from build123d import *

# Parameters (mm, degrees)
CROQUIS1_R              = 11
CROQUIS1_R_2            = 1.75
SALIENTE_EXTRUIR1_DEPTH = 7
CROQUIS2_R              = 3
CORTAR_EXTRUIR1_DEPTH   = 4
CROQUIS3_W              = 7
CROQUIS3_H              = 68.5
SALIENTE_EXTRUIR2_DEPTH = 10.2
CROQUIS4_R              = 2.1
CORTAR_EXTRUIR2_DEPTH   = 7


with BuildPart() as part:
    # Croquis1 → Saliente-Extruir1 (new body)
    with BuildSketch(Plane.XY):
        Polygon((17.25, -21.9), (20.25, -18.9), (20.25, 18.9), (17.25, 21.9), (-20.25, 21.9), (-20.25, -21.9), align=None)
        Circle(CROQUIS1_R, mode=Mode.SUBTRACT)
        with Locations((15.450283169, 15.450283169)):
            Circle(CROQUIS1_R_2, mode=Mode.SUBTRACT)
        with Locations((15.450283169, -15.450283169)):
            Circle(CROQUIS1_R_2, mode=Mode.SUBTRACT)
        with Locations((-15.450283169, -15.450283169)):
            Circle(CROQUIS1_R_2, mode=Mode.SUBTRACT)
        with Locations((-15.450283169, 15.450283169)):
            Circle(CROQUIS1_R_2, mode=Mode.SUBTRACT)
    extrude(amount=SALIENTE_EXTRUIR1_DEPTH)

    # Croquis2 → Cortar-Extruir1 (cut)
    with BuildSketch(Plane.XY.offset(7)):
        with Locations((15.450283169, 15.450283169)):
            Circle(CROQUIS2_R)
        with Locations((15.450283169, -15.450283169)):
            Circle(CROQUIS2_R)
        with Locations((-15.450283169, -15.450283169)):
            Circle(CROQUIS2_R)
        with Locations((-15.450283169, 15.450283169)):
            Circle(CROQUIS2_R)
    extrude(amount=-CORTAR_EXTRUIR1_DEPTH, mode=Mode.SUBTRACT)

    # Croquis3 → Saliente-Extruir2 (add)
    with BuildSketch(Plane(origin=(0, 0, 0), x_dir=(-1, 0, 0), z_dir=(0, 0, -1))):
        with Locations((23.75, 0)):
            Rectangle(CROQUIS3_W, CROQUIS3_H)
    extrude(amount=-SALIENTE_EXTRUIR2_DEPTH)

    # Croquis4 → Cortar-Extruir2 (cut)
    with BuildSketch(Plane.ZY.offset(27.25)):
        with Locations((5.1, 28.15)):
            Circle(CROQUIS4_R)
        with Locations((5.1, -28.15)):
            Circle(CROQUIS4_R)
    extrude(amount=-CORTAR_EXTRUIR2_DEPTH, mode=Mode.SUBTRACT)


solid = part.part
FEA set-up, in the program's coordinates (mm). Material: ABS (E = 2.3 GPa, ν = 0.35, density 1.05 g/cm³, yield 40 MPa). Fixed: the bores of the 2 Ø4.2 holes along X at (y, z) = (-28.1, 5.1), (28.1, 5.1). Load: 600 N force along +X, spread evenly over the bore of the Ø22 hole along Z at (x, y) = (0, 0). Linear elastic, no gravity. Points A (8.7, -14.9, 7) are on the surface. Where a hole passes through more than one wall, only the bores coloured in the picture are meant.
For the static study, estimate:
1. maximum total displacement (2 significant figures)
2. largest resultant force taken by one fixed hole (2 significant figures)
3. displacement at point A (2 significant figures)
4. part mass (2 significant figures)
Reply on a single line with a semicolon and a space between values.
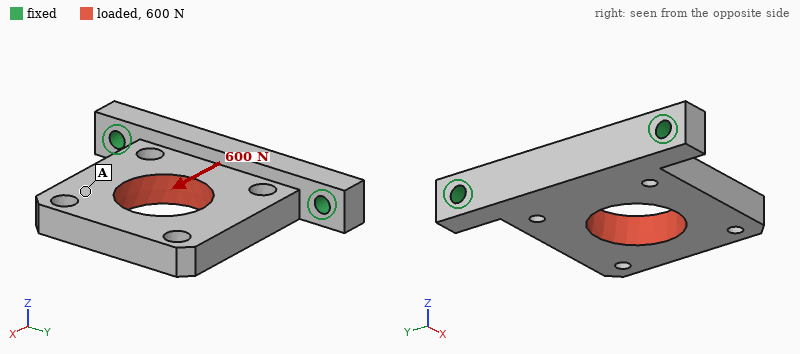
0.27 mm; 330 N; 0.20 mm; 15 g
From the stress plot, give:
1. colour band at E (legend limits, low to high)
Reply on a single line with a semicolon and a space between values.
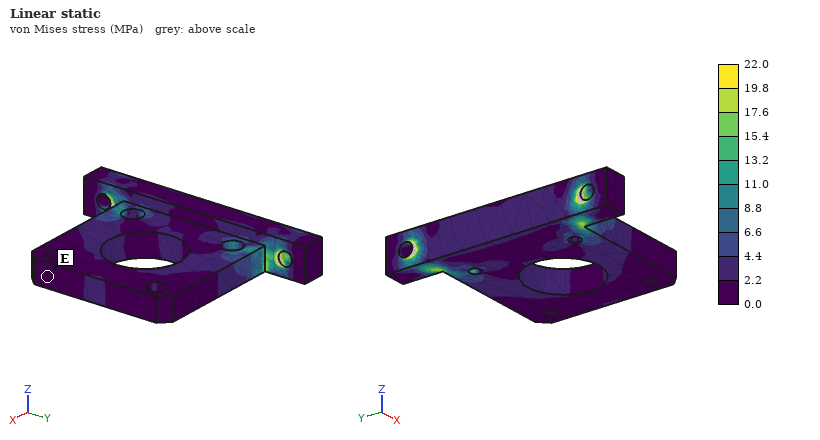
0.0 to 2.2 MPa
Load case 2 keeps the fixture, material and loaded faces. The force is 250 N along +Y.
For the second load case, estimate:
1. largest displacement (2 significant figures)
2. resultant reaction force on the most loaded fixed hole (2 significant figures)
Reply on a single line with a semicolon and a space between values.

0.17 mm; 180 N
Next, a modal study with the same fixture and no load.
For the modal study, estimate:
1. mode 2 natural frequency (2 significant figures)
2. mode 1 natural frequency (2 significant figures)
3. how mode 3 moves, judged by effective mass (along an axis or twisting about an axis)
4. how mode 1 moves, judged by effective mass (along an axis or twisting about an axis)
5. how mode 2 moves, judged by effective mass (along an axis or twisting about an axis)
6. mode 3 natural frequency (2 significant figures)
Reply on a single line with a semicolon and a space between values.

1600 Hz; 530 Hz; along Y; along Z; twisting about X; 2300 Hz
